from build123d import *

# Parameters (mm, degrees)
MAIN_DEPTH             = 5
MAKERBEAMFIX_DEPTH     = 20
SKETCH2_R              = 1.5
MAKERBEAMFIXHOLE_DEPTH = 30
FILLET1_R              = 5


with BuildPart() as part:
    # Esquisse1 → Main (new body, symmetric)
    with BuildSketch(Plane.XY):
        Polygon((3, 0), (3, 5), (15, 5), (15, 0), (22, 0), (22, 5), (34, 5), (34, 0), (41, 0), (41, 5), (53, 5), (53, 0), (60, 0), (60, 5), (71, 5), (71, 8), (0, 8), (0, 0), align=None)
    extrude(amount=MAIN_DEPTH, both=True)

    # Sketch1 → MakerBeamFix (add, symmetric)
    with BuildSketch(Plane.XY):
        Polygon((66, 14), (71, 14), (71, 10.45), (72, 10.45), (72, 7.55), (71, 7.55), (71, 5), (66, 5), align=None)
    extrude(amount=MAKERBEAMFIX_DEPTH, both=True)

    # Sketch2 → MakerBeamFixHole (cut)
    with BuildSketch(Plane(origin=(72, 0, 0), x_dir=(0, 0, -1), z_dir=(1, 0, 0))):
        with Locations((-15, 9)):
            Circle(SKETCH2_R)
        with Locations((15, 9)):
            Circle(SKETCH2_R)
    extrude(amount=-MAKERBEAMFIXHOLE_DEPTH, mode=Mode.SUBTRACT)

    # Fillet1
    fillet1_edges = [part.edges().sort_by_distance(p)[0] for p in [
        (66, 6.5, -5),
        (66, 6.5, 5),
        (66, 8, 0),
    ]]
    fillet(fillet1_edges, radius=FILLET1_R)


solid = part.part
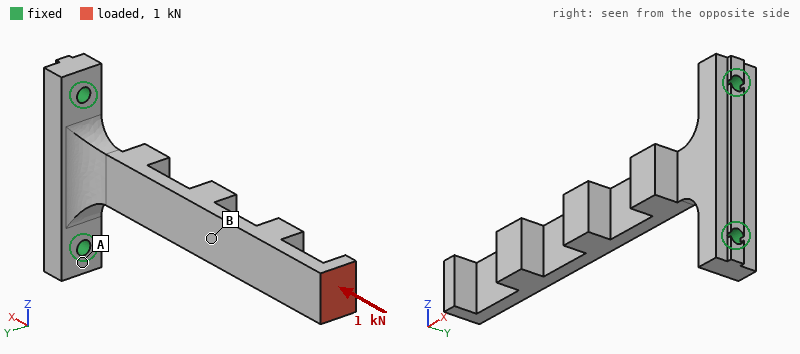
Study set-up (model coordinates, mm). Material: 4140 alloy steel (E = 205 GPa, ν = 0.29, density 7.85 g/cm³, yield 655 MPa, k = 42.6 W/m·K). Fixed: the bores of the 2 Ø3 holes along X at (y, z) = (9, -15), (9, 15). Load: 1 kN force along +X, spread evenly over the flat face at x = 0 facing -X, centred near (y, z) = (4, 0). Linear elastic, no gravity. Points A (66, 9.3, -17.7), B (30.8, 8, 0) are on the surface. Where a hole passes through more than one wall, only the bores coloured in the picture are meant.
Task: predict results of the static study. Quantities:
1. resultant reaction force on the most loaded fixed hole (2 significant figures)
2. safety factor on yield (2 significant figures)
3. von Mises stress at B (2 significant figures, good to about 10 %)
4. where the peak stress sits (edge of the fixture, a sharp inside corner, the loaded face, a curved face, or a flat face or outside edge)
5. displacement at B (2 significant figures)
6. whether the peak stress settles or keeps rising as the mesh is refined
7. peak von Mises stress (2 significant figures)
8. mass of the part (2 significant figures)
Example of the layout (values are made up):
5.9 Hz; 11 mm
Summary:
560 N; 2.8; 120 MPa; a curved face; 0.27 mm; settles; 240 MPa; 40 g
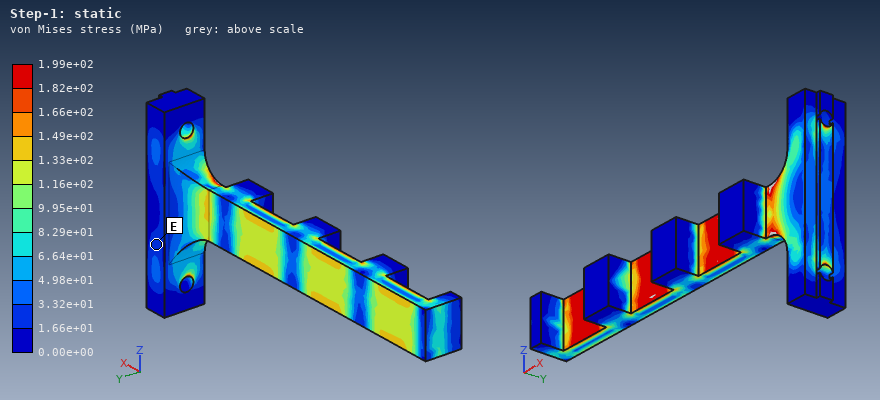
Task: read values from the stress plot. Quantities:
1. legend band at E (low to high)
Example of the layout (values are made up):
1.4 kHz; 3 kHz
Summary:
1.66e+01 to 3.32e+01 MPa
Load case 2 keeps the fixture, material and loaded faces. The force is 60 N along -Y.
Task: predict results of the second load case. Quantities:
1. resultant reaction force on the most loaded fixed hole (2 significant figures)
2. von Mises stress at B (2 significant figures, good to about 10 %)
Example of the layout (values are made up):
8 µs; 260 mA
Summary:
44 N; 120 MPa
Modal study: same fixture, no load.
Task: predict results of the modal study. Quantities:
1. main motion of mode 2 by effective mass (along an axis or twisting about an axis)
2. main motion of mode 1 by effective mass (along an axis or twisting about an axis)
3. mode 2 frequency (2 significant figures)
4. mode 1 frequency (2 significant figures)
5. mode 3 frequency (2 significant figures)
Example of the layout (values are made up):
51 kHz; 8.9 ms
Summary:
along Z; along Y; 1500 Hz; 520 Hz; 3000 Hz
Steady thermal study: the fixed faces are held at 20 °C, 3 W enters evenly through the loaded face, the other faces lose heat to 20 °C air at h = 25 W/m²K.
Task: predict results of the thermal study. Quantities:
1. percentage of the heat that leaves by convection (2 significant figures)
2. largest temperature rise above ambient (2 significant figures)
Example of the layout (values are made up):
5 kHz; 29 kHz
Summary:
66 %; 81 K
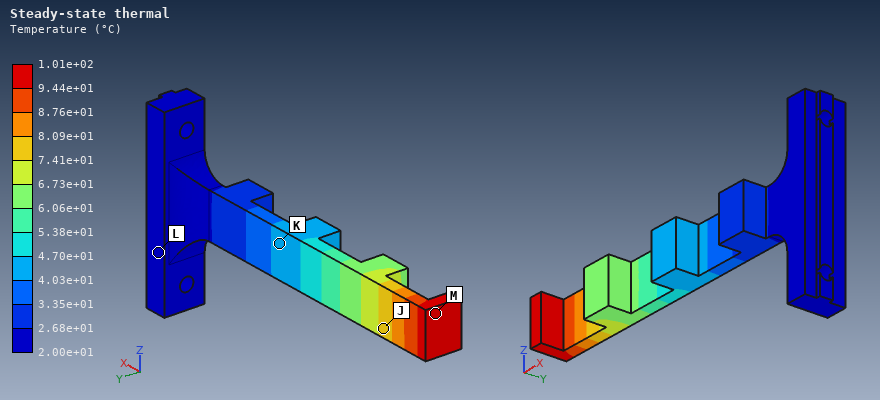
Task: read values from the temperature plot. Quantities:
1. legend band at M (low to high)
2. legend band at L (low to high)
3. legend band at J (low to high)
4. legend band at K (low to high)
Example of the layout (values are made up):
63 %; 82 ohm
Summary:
9.44e+01 to 1.01e+02 °C; 2.00e+01 to 2.68e+01 °C; 7.41e+01 to 8.09e+01 °C; 4.03e+01 to 4.70e+01 °C
